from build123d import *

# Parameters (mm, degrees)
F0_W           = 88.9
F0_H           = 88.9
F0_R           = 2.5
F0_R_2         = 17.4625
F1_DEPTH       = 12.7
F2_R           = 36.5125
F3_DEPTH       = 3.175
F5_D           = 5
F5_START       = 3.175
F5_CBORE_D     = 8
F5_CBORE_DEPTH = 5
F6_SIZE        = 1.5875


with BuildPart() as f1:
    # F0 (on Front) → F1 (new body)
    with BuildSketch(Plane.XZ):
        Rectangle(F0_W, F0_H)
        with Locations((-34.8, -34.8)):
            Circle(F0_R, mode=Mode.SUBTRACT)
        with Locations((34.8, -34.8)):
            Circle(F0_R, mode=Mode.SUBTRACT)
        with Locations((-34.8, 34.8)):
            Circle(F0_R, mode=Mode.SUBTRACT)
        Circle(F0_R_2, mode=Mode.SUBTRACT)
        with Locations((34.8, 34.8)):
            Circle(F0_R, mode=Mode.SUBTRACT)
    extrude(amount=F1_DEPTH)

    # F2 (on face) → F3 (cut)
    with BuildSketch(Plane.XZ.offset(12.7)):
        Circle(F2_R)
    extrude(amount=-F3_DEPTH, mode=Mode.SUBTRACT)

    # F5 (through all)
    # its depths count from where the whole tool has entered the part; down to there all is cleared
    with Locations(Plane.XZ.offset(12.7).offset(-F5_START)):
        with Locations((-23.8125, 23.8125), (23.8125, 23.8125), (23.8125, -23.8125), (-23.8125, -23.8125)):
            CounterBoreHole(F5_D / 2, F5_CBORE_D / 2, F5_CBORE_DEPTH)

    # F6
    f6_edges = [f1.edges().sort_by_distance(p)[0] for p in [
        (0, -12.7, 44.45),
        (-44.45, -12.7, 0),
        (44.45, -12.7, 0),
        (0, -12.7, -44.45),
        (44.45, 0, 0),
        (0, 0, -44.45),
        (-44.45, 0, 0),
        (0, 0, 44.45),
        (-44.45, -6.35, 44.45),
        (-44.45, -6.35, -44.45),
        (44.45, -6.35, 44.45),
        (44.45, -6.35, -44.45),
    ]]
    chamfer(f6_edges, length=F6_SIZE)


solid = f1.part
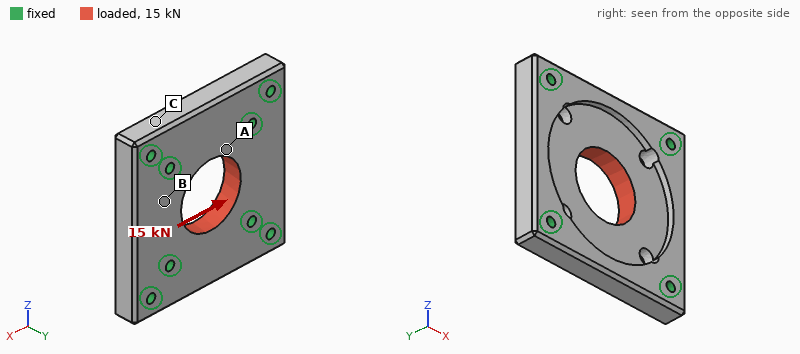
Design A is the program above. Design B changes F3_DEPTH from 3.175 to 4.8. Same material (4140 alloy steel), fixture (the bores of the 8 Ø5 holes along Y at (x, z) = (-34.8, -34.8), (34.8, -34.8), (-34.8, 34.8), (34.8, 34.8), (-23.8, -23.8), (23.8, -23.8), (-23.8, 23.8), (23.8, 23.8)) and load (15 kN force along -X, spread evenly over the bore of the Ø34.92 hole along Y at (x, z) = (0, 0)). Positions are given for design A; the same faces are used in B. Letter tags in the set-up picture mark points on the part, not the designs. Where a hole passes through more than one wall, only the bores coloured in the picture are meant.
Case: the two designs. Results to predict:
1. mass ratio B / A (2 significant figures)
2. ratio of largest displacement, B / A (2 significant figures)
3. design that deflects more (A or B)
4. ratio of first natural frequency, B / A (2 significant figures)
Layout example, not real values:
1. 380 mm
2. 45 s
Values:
1. 0.93
2. 1.1
3. B
4. 0.99
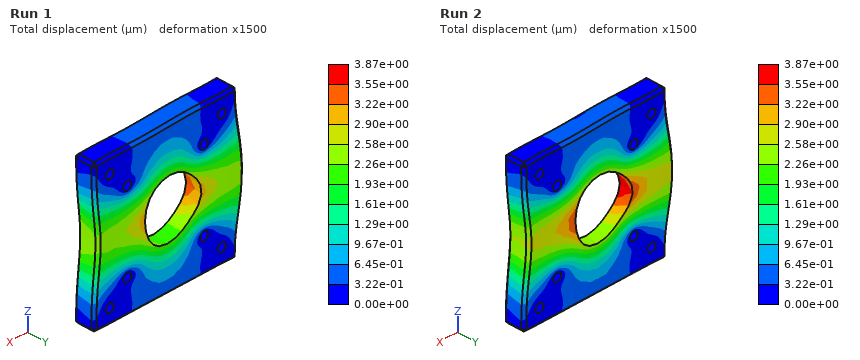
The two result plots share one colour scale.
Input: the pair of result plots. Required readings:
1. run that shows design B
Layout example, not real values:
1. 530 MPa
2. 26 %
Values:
1. Run 2
